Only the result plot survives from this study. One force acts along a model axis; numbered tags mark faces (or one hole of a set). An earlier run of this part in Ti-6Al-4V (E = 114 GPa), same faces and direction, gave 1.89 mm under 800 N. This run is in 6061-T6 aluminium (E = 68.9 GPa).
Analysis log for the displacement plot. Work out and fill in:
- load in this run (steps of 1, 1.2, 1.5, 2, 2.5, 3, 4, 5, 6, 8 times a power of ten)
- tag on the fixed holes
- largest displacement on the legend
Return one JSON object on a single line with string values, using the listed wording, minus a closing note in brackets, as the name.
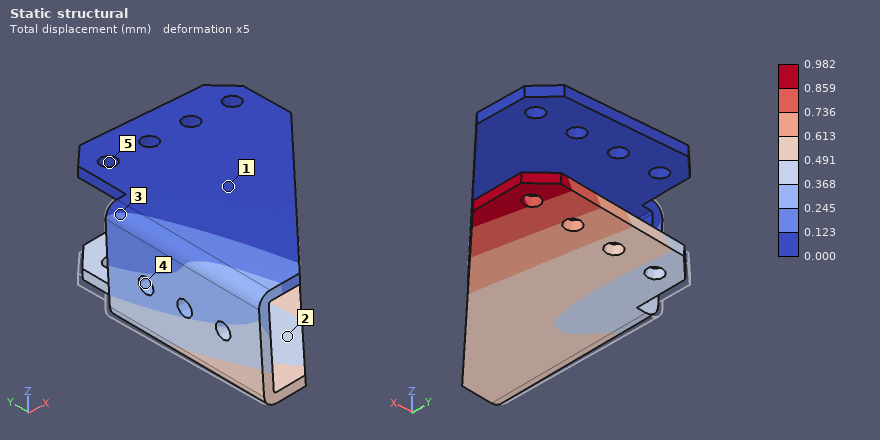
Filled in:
{"load in this run": "250 N", "tag on the fixed holes": "5", "largest displacement on the legend": "0.982 mm"}
